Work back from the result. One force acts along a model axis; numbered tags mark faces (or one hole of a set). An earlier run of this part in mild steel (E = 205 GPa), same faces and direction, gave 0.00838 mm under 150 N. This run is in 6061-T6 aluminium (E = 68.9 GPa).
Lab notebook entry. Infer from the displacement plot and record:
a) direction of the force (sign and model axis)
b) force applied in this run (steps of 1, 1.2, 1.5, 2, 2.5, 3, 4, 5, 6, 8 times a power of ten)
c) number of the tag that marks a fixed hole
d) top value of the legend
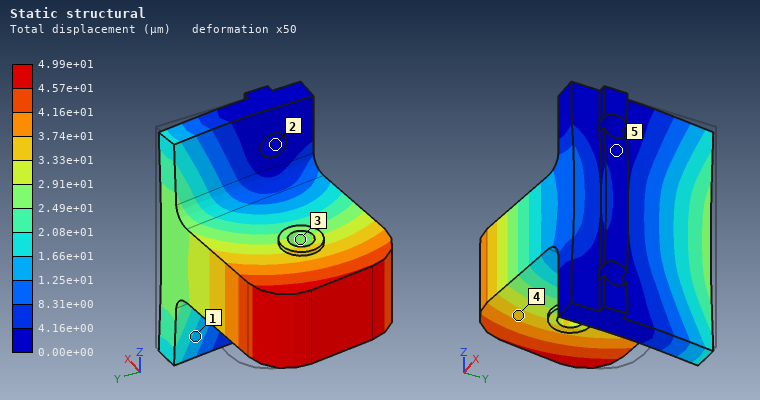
-Y
300 N
2
4.99e+01 µm
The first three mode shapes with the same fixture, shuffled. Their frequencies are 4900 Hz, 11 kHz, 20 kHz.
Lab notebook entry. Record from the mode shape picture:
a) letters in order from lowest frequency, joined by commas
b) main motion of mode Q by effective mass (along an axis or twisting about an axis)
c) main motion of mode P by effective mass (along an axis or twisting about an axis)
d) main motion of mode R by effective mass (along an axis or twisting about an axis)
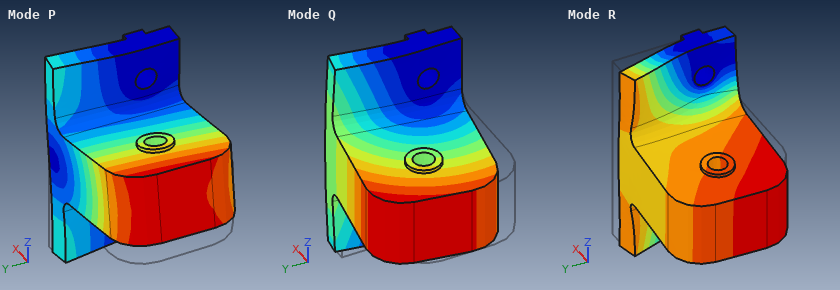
Q, P, R
along Y
along Z
along X
